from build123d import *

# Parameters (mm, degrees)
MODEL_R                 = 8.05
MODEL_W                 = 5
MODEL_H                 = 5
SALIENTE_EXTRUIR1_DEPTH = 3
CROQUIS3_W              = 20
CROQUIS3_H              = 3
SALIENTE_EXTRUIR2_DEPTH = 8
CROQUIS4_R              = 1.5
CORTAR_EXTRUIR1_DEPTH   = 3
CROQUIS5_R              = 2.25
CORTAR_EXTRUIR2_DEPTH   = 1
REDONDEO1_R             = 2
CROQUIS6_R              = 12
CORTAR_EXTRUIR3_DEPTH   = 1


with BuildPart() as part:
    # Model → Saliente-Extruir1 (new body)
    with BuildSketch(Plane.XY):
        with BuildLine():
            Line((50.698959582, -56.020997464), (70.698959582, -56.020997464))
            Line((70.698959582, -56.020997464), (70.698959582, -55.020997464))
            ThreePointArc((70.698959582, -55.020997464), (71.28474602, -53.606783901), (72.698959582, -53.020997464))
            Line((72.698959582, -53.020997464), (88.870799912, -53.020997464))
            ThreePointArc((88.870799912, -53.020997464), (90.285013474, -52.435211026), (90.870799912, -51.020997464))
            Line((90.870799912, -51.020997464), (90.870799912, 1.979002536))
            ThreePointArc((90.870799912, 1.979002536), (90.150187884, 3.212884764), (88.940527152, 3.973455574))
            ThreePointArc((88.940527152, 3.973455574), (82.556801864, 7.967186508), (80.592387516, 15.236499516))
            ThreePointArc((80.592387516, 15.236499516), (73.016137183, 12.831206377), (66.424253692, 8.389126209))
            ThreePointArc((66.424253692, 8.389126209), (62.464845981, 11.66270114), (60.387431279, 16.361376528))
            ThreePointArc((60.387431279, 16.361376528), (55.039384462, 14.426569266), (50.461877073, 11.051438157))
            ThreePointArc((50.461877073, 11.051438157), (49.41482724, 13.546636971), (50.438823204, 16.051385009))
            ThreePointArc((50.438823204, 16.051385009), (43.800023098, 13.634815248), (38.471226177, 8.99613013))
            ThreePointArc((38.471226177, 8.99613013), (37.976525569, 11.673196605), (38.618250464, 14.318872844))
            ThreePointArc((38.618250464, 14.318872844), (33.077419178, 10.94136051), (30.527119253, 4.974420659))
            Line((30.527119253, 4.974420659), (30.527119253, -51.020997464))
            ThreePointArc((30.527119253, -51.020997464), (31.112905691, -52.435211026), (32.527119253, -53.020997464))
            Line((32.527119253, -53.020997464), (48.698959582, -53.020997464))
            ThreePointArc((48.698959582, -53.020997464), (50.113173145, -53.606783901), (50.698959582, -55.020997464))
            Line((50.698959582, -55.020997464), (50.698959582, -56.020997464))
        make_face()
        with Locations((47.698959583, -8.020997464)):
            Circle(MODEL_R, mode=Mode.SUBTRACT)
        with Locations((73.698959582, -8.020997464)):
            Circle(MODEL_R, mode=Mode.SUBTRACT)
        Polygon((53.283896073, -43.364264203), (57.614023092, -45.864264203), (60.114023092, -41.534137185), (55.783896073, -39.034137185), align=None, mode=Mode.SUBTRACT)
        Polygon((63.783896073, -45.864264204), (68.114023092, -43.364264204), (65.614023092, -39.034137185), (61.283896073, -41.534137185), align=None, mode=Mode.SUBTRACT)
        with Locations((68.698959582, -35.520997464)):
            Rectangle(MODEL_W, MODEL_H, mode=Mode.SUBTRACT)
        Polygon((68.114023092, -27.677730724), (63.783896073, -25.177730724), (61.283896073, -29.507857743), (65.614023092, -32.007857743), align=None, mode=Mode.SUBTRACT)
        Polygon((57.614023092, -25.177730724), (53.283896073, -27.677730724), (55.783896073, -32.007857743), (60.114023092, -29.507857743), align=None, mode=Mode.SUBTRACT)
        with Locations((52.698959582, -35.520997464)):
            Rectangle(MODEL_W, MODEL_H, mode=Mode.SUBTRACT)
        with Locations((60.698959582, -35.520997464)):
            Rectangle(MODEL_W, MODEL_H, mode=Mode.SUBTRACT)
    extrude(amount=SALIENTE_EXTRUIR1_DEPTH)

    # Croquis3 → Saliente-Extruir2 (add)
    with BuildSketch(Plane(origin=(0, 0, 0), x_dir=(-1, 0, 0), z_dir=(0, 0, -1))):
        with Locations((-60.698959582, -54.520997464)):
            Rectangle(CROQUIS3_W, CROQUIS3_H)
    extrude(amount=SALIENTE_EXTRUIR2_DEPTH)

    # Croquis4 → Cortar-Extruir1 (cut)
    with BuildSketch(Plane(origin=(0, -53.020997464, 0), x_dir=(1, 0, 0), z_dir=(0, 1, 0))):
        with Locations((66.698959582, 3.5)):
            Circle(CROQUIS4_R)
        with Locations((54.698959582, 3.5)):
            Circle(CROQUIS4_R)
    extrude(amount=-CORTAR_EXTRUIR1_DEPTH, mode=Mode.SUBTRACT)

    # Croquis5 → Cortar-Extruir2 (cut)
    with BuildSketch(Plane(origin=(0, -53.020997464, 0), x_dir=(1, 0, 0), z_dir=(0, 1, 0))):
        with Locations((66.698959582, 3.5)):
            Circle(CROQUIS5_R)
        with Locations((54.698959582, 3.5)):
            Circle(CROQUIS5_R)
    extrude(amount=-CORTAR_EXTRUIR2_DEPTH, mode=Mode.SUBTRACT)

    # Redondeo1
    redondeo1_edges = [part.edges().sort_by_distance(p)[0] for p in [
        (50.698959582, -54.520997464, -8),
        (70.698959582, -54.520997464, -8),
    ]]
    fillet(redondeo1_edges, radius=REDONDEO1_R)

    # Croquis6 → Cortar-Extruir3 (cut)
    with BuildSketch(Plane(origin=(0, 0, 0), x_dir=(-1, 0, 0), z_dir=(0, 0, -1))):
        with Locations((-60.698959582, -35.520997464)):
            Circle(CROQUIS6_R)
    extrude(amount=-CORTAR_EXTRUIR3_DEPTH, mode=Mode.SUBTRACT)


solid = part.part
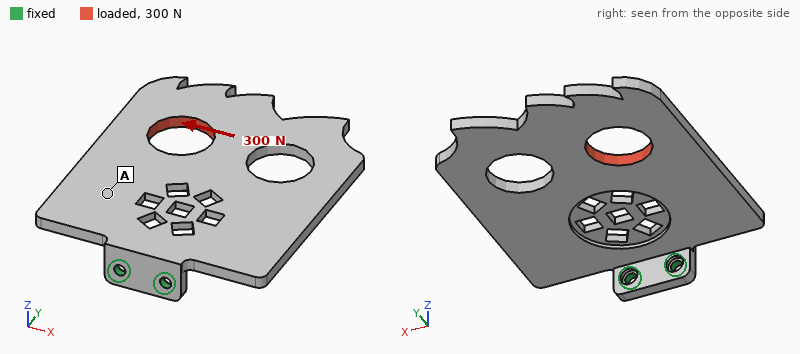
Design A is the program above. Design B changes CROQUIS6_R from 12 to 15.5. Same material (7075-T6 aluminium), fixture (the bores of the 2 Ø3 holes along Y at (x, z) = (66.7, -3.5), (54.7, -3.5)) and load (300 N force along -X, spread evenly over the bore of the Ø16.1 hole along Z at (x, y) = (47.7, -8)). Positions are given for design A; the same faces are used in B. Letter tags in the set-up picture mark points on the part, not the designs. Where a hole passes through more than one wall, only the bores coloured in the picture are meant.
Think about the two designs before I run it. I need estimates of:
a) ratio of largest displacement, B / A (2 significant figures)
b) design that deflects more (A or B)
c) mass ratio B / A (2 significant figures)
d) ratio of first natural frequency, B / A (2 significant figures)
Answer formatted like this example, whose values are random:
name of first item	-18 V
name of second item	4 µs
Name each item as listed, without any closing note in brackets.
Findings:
ratio of largest displacement, B / A	1.1
design that deflects more	B
mass ratio B / A	0.97
ratio of first natural frequency, B / A	0.93
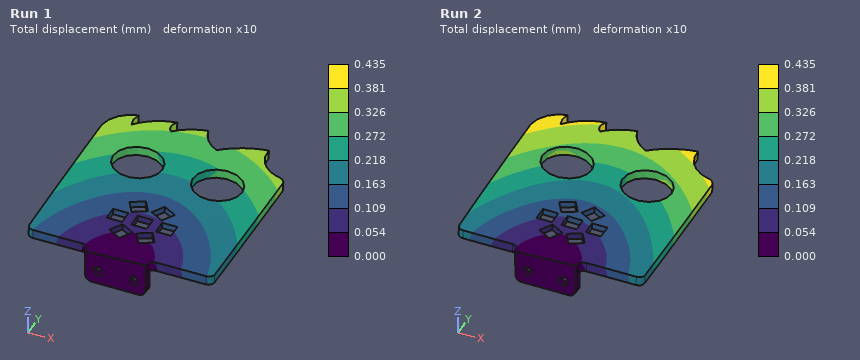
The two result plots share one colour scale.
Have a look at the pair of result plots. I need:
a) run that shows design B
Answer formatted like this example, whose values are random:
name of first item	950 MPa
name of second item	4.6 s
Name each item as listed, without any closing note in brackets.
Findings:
run that shows design B	Run 2
